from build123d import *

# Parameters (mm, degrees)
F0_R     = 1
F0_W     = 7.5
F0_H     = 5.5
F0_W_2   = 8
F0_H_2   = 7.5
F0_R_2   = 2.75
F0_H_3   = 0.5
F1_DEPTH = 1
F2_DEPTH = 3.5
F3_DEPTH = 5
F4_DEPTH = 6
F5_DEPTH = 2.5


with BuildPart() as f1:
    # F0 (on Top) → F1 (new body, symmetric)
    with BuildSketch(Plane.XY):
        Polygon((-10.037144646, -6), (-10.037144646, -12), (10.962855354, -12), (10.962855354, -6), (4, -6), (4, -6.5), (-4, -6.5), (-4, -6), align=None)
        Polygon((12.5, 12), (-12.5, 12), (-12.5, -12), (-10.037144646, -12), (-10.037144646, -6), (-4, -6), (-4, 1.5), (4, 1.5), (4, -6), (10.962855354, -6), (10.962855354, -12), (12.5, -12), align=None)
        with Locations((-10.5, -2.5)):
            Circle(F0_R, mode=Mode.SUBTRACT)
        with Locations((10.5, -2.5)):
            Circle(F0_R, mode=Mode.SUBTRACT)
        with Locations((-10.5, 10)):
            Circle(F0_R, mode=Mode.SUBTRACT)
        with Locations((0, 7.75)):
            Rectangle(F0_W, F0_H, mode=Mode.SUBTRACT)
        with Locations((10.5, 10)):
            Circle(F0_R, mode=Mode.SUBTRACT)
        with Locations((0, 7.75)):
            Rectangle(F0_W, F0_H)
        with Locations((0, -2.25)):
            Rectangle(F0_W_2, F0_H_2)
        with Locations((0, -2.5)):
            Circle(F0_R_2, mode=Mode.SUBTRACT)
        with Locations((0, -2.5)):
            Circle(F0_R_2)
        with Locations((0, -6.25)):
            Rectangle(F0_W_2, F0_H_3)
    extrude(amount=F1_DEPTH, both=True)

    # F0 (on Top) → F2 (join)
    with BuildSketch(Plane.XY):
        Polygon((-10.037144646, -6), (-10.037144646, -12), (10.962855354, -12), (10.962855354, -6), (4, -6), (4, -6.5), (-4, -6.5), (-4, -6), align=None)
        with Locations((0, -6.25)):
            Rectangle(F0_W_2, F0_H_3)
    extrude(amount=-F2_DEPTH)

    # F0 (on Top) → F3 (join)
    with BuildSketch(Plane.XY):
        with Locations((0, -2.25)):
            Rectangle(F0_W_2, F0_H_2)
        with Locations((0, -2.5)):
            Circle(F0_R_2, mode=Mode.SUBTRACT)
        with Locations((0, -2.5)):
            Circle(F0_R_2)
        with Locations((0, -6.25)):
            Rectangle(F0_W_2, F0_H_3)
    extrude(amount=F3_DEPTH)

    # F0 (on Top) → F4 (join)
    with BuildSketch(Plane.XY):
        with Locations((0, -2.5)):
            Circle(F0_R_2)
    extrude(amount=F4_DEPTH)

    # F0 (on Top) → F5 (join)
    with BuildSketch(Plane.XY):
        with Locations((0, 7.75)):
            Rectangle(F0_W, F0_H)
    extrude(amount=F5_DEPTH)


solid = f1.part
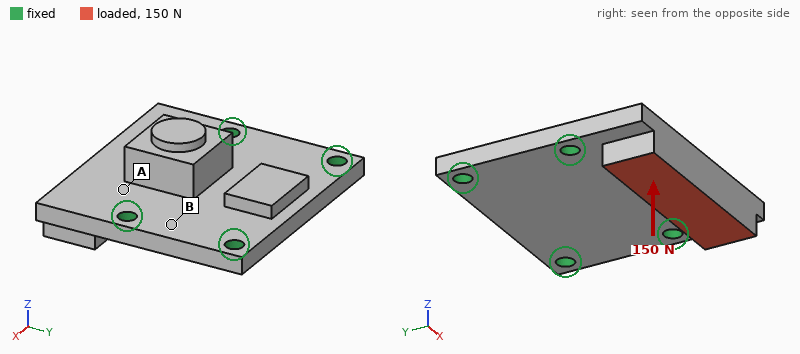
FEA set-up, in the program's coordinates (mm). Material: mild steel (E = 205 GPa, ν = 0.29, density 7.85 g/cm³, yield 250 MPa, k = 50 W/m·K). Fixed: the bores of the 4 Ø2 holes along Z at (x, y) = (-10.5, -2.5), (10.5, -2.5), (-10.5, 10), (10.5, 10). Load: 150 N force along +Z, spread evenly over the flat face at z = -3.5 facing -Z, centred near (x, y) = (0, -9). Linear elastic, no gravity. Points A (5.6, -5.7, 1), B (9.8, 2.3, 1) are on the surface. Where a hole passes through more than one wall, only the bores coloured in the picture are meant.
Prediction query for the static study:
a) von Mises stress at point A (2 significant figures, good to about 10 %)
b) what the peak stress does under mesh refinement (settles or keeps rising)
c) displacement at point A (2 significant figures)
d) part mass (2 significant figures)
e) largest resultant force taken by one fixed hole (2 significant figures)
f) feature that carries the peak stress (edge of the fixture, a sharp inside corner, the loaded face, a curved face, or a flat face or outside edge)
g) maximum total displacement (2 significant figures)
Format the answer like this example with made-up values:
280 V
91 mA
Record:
20 MPa
keeps rising
2.5 µm
14 g
95 N
edge of the fixture
8.0 µm
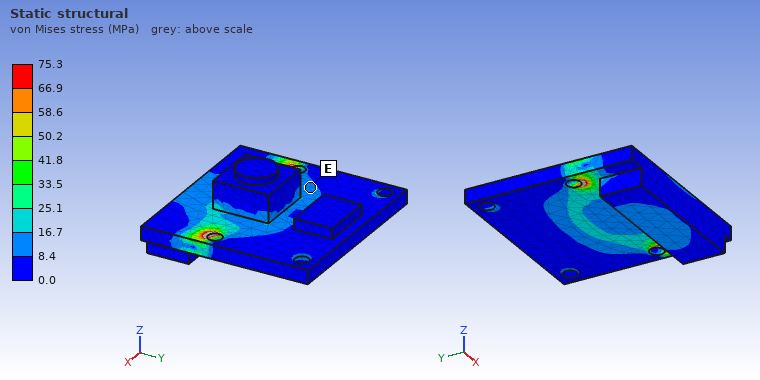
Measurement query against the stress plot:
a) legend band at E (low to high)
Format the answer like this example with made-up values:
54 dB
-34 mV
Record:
8.4 to 16.7 MPa
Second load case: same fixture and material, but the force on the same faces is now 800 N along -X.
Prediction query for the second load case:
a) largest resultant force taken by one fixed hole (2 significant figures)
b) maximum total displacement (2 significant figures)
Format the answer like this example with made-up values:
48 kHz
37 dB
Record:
450 N
5.3 µm
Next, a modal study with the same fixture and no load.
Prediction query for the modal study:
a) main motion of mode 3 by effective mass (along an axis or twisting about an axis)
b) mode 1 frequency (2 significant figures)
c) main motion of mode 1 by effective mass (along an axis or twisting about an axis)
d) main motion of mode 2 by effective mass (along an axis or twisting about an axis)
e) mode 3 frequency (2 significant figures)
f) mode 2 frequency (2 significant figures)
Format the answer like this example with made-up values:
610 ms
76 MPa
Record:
twisting about Y
11 kHz
along Z
along Z
28 kHz
21 kHz
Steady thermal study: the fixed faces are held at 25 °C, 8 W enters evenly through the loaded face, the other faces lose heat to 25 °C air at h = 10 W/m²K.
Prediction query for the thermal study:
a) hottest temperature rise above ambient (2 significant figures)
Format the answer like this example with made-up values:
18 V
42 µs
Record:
28 K
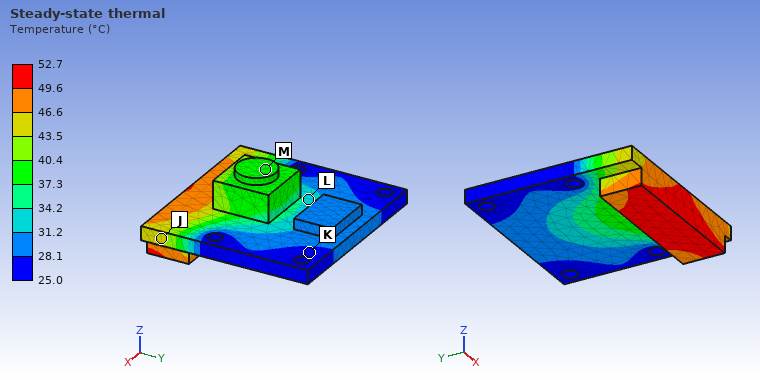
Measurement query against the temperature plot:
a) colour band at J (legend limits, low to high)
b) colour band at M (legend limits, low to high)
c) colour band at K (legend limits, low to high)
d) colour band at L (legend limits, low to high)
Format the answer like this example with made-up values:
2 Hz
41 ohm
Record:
43.5 to 46.6 °C
37.3 to 40.4 °C
25.0 to 28.1 °C
31.2 to 34.2 °C
